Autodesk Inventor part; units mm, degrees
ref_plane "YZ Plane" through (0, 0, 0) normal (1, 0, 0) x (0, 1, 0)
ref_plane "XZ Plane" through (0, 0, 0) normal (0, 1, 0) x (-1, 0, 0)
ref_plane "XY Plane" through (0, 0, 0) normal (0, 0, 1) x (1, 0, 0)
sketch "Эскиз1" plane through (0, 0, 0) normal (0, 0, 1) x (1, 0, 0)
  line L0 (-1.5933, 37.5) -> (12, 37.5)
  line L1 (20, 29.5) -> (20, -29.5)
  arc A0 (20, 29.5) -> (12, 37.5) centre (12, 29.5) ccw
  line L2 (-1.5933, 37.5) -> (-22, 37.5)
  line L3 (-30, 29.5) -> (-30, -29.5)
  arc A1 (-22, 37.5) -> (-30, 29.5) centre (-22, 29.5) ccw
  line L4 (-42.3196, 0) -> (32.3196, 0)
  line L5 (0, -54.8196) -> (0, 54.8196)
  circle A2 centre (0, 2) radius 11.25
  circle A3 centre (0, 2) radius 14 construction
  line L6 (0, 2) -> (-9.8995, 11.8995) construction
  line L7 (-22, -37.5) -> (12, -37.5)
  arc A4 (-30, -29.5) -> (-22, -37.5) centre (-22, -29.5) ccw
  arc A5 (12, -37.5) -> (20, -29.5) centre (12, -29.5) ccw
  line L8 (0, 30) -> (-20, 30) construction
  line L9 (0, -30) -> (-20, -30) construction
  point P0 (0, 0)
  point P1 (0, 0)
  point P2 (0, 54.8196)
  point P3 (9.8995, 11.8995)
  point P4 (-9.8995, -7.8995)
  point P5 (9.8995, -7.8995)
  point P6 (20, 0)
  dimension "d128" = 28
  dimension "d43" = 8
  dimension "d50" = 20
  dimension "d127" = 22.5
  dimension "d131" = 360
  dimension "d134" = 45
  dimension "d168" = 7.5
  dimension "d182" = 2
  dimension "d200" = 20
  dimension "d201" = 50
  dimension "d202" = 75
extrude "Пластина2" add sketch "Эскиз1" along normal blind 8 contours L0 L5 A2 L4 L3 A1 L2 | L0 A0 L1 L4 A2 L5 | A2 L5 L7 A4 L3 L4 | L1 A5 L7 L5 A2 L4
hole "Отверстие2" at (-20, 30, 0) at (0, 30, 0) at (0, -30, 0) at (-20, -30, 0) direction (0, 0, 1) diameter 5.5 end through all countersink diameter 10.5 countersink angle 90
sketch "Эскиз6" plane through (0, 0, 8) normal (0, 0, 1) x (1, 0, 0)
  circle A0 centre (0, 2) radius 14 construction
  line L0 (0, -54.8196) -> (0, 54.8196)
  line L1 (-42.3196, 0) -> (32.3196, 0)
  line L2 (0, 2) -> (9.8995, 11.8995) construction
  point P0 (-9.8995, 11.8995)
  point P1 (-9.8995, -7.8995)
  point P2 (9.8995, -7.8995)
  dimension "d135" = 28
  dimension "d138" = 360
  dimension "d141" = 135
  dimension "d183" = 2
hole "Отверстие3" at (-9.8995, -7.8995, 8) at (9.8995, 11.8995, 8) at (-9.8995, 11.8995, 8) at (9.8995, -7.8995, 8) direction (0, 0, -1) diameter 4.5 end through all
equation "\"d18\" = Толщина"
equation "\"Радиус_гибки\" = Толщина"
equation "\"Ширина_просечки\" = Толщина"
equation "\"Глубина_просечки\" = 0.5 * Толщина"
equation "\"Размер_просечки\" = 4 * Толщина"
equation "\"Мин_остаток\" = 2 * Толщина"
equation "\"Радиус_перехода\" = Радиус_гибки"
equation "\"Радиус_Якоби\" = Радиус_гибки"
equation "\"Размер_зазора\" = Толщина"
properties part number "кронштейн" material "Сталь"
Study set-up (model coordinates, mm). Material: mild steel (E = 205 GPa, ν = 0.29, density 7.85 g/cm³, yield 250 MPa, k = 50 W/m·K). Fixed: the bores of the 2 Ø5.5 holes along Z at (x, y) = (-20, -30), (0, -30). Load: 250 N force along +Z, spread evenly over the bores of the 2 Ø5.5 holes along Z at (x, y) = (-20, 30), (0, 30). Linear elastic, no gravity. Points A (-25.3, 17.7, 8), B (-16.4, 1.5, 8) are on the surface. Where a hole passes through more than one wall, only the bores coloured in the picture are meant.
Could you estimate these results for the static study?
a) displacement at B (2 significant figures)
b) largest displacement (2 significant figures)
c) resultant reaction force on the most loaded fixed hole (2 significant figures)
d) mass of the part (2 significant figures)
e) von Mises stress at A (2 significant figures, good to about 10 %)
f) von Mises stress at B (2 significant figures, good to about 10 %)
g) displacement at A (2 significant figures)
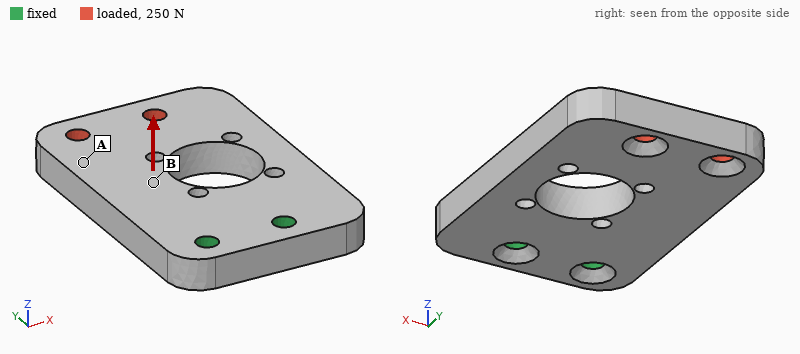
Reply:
23 µm
78 µm
140 N
190 g
9.3 MPa
24 MPa
46 µm
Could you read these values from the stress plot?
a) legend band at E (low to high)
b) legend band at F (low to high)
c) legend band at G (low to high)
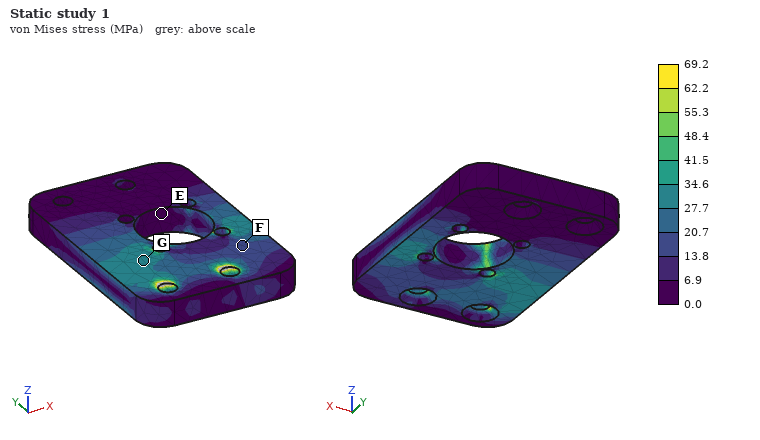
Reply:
0.0 to 6.9 MPa
13.8 to 20.7 MPa
27.7 to 34.6 MPa
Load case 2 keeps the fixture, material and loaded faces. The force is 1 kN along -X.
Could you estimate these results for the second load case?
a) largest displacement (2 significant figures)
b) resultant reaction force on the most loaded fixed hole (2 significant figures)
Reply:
21 µm
2.5 kN
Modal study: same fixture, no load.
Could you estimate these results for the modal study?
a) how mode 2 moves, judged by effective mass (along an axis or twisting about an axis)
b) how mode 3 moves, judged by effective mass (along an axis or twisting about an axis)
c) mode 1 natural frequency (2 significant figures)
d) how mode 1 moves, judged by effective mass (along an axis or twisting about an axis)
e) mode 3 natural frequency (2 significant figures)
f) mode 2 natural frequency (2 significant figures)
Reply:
twisting about Y
along X
1300 Hz
along Z
4400 Hz
3400 Hz
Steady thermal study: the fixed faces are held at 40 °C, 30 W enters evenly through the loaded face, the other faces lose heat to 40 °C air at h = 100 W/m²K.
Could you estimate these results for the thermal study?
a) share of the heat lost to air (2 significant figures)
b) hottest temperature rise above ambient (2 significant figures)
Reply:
74 %
66 K
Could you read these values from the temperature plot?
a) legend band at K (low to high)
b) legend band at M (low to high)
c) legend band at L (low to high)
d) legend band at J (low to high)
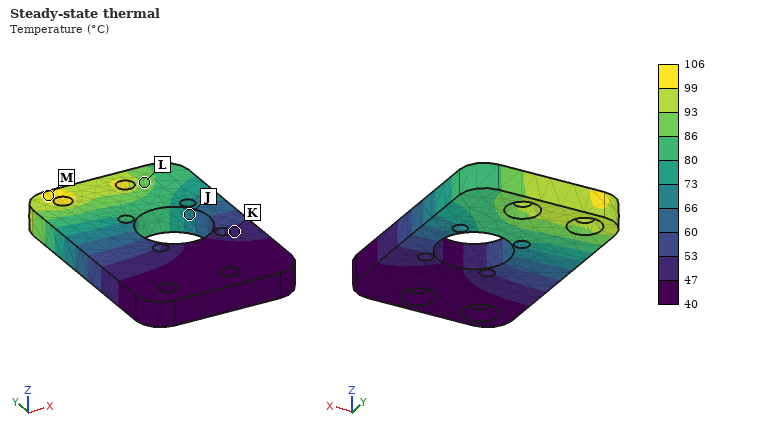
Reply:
47 to 53 °C
99 to 106 °C
86 to 93 °C
66 to 73 °C
